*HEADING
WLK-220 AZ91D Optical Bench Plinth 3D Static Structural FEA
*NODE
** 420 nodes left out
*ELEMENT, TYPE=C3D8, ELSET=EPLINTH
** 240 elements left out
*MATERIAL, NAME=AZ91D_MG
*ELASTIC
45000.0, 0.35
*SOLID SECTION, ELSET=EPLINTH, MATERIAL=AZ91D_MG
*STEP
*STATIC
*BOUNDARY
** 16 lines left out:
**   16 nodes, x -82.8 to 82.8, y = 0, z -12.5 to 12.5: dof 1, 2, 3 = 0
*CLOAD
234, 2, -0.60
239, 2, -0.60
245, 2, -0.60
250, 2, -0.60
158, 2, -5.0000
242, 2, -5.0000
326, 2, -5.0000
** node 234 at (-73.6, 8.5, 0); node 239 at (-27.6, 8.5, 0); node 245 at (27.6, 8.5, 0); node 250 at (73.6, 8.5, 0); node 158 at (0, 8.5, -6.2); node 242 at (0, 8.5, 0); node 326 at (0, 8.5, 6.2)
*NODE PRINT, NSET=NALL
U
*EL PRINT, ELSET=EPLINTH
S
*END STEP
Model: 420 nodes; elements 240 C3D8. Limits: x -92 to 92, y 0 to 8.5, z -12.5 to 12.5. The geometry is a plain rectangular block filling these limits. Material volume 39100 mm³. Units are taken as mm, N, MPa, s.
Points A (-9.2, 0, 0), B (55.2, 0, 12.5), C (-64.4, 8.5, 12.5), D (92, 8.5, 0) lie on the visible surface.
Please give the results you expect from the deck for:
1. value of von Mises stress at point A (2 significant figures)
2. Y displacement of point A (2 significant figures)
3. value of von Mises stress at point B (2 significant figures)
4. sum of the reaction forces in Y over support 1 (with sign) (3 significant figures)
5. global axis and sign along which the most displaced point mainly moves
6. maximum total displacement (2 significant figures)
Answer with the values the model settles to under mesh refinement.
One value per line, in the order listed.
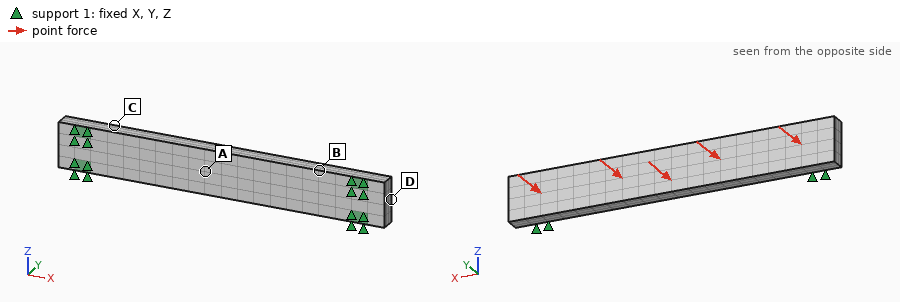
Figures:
0.71 MPa
-0.0054 mm
0.46 MPa
17.4 N
-Y
0.0058 mm
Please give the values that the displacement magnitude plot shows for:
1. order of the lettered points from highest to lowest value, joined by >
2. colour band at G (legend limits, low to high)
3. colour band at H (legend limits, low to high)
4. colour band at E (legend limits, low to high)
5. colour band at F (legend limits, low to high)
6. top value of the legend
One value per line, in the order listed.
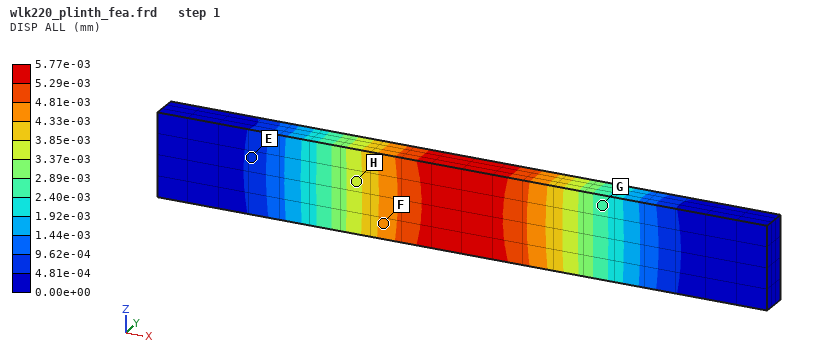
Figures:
F > H > G > E
2.40e-03 to 2.89e-03 mm
3.37e-03 to 3.85e-03 mm
4.81e-04 to 9.62e-04 mm
4.33e-03 to 4.81e-03 mm
5.77e-03 mm
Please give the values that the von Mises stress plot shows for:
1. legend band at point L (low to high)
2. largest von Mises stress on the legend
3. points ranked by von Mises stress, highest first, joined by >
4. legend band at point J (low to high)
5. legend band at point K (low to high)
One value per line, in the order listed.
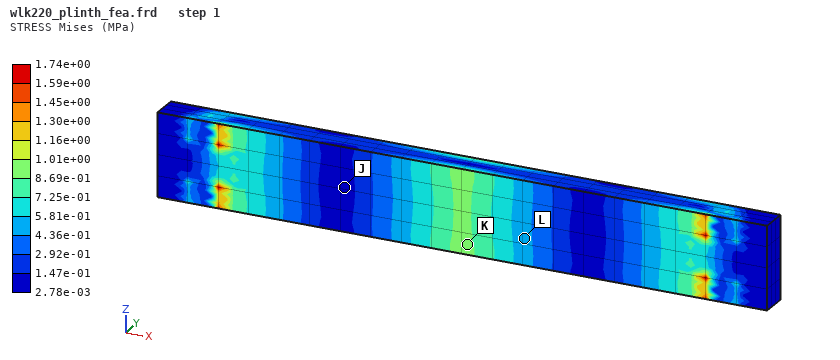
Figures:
4.36e-01 to 5.81e-01 MPa
1.74e+00 MPa
K > L > J
2.78e-03 to 1.47e-01 MPa
8.69e-01 to 1.01e+00 MPa
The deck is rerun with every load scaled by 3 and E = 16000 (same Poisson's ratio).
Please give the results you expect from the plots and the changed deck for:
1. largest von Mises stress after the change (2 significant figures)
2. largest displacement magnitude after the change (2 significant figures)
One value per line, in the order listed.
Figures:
5.2 MPa
0.049 mm
